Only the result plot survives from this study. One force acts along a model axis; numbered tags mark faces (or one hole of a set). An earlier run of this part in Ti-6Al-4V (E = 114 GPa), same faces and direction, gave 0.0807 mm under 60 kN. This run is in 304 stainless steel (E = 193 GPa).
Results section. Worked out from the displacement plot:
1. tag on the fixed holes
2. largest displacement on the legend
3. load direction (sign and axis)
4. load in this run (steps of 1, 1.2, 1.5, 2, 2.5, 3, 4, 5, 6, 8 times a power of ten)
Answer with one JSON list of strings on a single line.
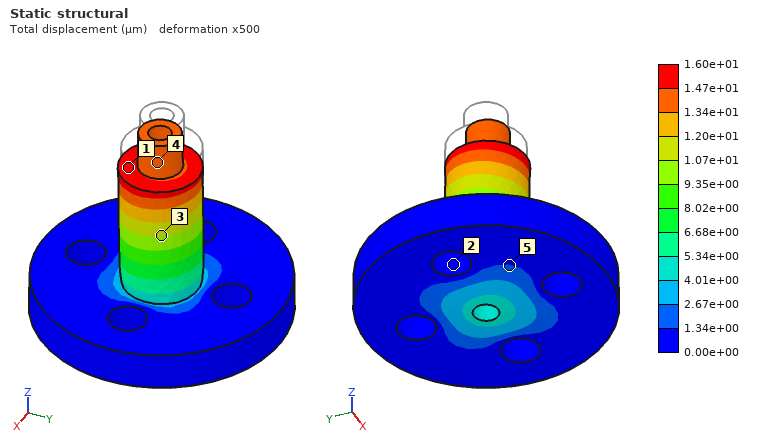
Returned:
["2", "1.60e+01 µm", "-Z", "20 kN"]
